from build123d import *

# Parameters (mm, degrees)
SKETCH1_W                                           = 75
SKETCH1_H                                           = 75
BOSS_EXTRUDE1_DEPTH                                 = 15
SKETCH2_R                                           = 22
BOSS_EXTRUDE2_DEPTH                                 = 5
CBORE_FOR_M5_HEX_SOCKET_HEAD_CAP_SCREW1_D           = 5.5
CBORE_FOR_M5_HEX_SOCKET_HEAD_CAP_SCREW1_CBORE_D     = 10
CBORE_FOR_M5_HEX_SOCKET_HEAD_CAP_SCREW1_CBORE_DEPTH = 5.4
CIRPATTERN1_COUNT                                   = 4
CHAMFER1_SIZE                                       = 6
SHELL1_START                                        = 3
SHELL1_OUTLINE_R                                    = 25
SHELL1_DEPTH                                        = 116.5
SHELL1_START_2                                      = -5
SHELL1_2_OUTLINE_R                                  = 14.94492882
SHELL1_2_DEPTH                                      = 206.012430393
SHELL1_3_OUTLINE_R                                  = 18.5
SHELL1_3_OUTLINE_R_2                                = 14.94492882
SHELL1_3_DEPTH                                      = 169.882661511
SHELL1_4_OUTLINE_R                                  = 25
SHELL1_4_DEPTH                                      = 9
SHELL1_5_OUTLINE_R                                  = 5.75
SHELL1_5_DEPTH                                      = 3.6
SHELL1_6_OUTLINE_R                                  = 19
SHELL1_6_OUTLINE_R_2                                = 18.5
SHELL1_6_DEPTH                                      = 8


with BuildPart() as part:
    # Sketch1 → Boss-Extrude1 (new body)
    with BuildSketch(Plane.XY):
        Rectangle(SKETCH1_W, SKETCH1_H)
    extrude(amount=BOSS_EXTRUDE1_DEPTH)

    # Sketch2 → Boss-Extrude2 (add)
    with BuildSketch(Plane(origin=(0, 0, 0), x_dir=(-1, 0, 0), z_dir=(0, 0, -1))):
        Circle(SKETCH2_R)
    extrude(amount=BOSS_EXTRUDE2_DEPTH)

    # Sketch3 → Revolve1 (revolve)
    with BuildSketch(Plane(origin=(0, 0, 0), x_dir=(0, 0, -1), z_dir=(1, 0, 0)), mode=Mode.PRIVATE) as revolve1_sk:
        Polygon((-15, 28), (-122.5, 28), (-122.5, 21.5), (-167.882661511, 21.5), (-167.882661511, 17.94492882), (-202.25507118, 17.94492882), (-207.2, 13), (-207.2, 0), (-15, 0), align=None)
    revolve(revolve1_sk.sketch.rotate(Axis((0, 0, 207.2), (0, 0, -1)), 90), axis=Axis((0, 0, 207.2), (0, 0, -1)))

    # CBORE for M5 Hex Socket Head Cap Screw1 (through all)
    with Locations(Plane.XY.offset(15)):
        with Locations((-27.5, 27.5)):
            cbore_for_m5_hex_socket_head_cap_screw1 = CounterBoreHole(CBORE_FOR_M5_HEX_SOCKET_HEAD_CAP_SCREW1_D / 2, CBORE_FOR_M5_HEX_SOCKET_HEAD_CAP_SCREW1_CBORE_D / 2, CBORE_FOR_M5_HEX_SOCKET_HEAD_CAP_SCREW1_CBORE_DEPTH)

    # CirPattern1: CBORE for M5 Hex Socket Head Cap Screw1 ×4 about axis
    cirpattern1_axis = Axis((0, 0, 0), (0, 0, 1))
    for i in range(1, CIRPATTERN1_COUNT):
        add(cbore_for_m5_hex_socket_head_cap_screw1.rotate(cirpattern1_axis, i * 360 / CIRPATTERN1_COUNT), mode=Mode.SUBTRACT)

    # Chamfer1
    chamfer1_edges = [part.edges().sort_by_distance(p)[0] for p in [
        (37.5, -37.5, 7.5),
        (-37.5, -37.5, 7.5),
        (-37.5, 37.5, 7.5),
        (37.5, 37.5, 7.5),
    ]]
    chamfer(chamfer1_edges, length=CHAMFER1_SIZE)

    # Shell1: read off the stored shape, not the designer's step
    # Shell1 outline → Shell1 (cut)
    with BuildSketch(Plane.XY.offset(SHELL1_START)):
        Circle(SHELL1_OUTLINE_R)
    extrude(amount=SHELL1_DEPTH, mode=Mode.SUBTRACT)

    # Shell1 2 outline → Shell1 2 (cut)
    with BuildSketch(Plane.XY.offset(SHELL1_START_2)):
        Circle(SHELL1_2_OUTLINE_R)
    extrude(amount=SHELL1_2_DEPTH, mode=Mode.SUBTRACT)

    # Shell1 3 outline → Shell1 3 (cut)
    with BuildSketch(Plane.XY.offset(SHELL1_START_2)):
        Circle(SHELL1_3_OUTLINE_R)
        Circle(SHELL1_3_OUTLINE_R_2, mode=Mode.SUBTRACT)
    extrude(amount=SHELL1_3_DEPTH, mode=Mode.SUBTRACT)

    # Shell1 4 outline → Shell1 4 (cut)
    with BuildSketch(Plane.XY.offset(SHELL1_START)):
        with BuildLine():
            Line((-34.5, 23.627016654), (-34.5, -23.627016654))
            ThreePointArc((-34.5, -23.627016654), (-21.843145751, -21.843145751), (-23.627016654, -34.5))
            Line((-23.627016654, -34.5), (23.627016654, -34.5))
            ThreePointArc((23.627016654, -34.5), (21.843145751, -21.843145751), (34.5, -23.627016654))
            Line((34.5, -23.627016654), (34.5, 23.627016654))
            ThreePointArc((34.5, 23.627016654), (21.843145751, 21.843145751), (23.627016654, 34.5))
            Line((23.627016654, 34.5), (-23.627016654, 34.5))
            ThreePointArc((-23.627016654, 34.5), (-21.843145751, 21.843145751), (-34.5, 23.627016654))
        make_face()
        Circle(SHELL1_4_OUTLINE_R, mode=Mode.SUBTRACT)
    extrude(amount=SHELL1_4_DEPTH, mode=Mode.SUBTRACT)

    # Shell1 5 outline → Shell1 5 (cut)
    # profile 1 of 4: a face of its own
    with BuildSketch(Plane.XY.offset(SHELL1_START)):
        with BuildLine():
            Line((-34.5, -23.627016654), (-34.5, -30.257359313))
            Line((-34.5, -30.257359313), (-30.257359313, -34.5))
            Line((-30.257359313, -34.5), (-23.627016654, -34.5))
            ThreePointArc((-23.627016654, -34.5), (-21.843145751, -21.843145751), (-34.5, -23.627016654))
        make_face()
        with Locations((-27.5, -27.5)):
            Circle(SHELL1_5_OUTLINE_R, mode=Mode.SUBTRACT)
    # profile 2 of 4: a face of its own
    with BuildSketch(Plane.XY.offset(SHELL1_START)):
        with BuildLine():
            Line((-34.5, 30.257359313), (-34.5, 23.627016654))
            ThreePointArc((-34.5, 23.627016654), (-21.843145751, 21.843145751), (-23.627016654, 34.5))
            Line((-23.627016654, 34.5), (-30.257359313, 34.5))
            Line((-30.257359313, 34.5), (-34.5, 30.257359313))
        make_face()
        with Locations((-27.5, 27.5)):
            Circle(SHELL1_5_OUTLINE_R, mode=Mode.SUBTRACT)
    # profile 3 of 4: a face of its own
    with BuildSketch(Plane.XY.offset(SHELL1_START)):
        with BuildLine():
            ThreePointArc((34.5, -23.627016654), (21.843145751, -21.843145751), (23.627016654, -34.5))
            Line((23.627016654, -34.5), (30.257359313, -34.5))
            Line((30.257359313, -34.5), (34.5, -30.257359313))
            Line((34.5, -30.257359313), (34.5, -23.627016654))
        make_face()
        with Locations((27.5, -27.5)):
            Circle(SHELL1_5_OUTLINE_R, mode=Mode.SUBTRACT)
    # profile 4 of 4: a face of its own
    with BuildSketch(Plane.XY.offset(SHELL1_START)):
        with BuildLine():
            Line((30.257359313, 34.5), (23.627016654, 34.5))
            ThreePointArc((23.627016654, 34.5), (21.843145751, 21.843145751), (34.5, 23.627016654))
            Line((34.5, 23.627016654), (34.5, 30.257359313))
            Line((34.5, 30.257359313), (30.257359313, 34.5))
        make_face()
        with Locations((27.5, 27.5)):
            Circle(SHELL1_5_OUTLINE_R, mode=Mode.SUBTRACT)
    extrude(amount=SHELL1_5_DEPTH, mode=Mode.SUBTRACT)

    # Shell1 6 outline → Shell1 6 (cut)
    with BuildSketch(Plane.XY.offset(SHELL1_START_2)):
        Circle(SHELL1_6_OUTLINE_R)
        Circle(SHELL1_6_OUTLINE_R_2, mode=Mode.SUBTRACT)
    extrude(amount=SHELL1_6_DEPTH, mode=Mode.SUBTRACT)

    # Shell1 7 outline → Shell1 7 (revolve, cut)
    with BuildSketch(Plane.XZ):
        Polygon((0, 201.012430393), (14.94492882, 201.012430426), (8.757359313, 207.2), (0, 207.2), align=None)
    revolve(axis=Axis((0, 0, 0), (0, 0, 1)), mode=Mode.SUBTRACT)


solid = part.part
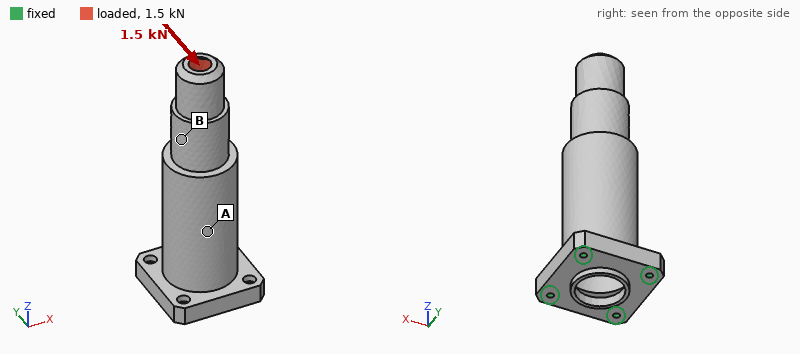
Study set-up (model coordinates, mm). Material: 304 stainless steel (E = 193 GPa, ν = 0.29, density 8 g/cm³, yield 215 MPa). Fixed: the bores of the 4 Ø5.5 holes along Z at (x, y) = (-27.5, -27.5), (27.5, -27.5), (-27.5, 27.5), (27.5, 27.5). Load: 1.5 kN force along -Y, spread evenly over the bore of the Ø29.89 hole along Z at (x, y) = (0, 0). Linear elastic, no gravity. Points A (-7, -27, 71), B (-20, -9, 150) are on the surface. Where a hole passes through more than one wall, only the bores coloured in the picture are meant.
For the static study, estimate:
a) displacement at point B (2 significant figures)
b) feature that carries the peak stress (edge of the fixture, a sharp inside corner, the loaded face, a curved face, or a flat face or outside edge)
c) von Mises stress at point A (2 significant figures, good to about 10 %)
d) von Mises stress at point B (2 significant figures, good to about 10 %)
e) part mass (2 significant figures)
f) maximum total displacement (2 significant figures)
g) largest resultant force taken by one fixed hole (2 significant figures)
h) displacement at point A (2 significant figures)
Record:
0.19 mm
a flat face or outside edge
27 MPa
13 MPa
990 g
0.30 mm
2.9 kN
0.072 mm
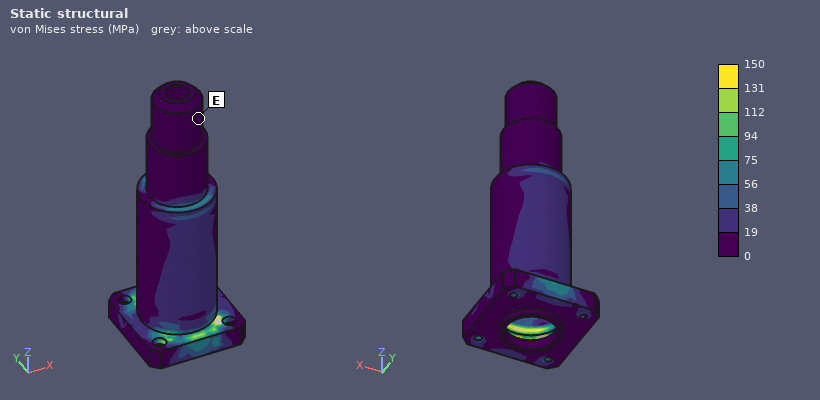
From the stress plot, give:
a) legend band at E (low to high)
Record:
0 to 19 MPa
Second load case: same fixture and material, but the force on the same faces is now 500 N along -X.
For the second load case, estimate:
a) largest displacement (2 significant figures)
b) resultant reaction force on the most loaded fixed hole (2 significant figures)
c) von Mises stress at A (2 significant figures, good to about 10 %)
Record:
99 µm
970 N
3.6 MPa
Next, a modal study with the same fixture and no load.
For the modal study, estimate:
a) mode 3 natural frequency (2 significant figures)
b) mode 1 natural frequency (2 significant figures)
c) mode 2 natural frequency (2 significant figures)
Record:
3800 Hz
800 Hz
800 Hz
